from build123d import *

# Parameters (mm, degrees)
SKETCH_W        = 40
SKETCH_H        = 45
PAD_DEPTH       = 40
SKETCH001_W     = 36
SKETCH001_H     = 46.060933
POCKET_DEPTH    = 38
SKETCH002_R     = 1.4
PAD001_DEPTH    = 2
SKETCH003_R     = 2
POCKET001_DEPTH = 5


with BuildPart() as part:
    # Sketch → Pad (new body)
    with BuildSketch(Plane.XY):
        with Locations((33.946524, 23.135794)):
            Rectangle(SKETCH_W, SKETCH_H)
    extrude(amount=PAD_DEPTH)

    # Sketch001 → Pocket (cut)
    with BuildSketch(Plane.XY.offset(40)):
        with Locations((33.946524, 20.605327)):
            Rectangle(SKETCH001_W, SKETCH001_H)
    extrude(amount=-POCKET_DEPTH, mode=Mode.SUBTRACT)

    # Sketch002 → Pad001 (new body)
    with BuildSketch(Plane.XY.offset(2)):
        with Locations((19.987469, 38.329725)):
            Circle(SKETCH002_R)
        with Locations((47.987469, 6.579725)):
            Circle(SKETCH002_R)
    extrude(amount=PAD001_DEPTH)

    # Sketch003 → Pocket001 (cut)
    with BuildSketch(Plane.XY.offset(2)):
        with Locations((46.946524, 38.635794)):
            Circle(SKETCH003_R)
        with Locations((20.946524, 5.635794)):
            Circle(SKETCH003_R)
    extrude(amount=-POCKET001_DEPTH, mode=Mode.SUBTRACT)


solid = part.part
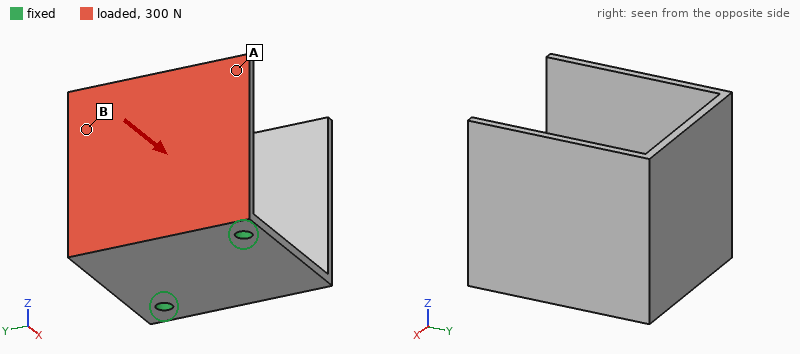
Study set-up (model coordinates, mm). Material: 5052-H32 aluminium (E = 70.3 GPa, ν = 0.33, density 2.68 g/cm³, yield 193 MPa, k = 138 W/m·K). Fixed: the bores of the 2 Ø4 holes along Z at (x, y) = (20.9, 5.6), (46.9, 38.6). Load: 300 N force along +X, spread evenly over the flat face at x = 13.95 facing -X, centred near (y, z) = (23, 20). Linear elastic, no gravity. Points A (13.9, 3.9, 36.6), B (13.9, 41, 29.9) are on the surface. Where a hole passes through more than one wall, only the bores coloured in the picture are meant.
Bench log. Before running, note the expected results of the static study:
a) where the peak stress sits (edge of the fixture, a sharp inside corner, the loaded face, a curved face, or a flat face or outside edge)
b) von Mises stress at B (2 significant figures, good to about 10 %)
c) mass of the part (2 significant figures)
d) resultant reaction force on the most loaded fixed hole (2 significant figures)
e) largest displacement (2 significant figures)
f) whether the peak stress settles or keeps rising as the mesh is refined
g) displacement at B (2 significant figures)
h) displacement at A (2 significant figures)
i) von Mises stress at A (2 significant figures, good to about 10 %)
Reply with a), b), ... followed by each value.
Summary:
a) edge of the fixture
b) 47 MPa
c) 35 g
d) 170 N
e) 0.83 mm
f) keeps rising
g) 0.29 mm
h) 0.72 mm
i) 16 MPa
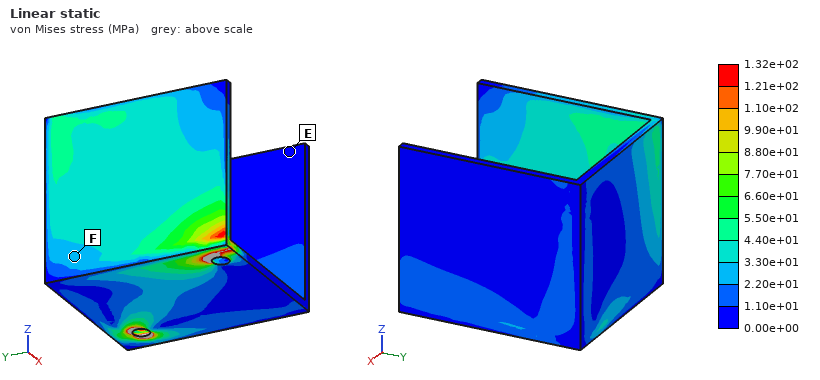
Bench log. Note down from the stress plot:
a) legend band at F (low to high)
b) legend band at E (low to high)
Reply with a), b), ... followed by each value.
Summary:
a) 2.20e+01 to 3.30e+01 MPa
b) 0.00e+00 to 1.10e+01 MPa
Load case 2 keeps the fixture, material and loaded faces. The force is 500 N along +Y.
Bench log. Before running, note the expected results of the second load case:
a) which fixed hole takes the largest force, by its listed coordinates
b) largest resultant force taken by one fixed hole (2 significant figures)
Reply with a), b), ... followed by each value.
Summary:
a) (20.9, 5.6)
b) 490 N
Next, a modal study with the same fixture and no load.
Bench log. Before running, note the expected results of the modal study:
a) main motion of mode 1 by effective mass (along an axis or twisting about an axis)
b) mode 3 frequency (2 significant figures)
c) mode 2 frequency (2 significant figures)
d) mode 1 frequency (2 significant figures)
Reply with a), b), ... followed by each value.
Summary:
a) along X
b) 1700 Hz
c) 1400 Hz
d) 950 Hz
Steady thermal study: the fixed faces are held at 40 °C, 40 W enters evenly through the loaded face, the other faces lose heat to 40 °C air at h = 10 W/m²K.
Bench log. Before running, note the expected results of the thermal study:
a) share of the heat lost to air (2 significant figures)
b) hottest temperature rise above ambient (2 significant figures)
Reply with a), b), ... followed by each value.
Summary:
a) 8.6 %
b) 80 K
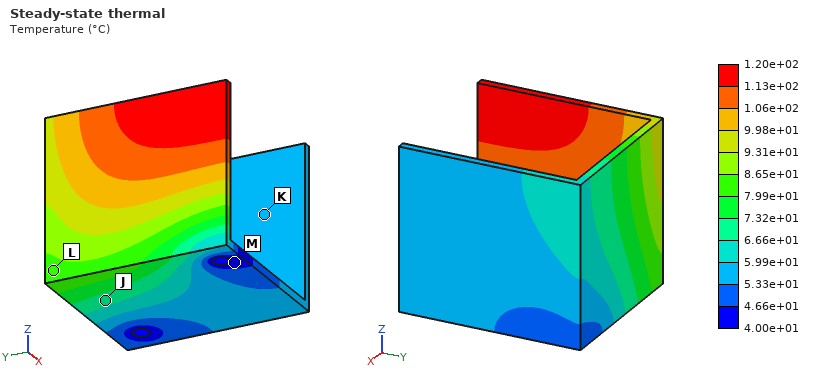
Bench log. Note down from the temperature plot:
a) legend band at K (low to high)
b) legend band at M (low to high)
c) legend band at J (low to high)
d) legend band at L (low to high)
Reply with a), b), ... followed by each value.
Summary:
a) 5.33e+01 to 5.99e+01 °C
b) 4.00e+01 to 4.66e+01 °C
c) 6.66e+01 to 7.32e+01 °C
d) 7.99e+01 to 8.65e+01 °C
